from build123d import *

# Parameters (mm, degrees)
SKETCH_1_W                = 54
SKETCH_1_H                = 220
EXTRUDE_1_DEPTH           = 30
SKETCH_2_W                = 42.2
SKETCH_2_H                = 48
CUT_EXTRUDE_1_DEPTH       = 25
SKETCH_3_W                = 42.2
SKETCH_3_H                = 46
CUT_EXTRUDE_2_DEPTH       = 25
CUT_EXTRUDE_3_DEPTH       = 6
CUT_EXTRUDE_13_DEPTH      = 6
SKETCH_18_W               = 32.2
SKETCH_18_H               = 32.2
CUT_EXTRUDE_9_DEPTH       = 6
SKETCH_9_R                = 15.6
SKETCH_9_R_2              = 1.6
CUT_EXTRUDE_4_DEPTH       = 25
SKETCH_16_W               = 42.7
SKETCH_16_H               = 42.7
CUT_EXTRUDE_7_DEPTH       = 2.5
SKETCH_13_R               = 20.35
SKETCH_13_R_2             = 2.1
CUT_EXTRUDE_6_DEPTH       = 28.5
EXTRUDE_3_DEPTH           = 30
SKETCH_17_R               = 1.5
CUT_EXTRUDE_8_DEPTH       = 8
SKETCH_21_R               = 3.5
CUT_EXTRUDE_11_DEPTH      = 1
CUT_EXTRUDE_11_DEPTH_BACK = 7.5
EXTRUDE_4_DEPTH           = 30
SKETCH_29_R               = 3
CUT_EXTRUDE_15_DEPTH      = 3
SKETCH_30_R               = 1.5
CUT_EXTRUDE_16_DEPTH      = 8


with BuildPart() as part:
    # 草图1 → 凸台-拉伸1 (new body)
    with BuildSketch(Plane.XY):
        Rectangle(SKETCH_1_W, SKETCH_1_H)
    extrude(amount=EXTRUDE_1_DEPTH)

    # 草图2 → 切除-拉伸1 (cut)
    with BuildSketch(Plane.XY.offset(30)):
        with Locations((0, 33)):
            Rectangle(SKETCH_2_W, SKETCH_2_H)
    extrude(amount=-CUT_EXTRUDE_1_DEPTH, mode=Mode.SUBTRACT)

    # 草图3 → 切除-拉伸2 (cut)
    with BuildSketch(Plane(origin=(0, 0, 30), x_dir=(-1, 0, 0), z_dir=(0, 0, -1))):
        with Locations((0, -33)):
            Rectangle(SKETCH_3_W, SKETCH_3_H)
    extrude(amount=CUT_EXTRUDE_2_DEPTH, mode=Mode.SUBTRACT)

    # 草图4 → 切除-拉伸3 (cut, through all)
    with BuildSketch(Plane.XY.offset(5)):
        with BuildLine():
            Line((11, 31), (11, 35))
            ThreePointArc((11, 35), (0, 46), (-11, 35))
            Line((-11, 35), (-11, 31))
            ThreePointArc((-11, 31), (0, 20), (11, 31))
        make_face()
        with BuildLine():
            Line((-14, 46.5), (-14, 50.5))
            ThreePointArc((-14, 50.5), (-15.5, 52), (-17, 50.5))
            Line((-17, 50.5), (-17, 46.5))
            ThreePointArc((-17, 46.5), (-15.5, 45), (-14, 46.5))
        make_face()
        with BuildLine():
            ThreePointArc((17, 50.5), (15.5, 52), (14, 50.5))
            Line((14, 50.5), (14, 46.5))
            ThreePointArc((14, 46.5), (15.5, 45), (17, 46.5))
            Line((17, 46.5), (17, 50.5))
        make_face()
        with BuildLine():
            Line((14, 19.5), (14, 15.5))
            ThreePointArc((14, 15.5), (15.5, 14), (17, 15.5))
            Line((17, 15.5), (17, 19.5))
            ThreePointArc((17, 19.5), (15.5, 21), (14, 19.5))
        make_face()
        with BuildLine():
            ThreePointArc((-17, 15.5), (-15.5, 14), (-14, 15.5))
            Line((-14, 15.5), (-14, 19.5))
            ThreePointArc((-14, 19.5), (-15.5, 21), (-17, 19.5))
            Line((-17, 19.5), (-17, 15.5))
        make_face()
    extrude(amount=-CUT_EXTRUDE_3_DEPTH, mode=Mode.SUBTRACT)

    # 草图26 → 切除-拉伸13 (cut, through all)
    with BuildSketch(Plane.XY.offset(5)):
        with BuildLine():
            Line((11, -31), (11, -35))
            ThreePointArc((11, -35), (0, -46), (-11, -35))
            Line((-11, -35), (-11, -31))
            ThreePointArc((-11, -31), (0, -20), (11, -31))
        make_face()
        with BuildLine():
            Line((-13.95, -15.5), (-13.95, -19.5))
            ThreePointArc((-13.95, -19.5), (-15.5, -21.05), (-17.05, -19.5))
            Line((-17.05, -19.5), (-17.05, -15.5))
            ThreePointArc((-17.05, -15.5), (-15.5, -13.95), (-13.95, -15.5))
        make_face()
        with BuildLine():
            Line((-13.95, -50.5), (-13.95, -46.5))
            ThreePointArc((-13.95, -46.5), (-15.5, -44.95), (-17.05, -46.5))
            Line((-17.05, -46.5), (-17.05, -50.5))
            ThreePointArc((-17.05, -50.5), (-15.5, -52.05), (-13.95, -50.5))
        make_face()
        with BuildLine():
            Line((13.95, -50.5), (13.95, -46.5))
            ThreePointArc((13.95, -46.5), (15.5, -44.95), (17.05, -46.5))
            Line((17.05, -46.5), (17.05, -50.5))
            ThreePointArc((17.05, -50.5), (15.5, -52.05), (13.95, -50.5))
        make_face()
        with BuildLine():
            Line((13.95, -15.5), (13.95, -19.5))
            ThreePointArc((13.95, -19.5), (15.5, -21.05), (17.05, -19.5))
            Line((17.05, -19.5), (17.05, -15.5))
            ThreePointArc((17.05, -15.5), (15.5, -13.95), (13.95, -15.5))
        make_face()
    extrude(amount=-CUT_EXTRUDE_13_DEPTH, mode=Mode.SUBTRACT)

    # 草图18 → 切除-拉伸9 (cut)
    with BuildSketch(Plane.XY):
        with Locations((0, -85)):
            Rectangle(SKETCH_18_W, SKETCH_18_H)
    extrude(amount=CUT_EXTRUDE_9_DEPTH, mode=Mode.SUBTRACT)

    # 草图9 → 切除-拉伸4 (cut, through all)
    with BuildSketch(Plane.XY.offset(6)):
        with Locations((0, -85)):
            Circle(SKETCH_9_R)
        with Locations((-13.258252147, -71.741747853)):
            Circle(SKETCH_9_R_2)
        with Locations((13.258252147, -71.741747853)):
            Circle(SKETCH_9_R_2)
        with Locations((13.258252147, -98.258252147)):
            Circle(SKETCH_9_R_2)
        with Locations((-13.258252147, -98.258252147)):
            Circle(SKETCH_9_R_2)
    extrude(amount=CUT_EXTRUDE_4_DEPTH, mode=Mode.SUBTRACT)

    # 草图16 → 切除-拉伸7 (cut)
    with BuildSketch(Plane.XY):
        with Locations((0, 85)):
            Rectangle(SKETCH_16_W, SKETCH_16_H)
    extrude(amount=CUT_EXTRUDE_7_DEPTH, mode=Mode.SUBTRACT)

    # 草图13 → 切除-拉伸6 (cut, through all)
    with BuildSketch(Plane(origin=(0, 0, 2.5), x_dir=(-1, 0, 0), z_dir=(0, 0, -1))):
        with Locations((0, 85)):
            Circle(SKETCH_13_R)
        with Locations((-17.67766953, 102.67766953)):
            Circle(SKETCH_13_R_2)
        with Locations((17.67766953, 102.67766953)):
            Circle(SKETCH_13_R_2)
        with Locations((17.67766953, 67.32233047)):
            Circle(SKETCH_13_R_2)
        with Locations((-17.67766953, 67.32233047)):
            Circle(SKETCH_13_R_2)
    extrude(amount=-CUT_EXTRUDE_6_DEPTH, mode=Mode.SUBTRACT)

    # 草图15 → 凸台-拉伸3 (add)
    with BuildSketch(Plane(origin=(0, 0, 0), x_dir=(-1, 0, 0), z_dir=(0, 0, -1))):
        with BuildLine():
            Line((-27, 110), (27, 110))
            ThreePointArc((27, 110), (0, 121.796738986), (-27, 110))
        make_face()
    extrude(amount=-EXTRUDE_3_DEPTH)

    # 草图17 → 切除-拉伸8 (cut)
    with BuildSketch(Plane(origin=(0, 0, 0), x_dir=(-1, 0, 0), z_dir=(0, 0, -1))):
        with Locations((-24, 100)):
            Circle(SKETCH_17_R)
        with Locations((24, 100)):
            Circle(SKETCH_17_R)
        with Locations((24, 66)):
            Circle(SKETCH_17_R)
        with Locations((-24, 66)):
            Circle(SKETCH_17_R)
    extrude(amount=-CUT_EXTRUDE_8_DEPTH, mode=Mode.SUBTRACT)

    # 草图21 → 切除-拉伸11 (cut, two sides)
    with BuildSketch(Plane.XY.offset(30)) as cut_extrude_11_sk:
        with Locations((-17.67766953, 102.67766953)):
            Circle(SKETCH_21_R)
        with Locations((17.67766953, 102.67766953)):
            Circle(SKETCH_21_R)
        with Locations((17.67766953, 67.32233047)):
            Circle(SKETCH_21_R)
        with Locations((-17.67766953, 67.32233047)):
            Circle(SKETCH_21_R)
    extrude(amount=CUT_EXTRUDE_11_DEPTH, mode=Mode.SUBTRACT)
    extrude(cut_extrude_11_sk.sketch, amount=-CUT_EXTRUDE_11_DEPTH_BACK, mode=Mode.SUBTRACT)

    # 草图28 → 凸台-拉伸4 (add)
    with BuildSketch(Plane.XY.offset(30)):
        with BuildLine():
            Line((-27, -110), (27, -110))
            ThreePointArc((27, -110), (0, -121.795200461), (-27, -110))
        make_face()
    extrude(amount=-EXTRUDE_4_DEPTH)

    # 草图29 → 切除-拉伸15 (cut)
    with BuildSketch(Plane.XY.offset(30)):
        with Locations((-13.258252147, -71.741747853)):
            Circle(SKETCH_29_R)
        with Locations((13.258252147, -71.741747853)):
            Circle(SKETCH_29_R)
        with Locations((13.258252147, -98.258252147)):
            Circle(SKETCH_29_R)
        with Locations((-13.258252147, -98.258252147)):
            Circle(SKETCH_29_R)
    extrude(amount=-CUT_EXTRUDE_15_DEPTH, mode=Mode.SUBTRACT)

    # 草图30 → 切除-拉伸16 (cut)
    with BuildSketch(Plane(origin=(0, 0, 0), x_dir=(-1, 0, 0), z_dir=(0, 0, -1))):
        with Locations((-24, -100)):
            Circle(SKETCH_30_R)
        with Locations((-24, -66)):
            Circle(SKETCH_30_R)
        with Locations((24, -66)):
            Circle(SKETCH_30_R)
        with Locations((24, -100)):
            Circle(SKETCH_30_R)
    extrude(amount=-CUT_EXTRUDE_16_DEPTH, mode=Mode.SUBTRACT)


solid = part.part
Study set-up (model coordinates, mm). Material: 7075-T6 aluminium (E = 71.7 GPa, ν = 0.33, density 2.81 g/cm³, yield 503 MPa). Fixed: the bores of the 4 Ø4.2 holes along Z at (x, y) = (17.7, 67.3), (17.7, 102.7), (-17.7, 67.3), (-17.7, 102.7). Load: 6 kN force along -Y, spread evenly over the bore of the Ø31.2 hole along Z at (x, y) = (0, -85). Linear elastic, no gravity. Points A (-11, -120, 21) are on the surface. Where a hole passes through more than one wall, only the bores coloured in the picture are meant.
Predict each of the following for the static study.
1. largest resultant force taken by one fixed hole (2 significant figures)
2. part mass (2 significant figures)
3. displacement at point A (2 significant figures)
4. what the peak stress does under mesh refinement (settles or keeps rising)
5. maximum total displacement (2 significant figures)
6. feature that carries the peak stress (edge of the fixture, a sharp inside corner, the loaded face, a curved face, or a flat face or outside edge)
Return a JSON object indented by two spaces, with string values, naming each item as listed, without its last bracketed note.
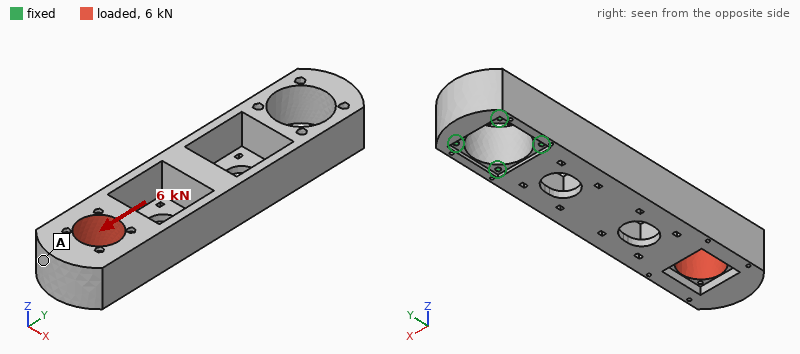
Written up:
{
  "largest resultant force taken by one fixed hole": "2.4 kN",
  "part mass": "590 g",
  "displacement at point A": "0.22 mm",
  "what the peak stress does under mesh refinement": "keeps rising",
  "maximum total displacement": "0.23 mm",
  "feature that carries the peak stress": "edge of the fixture"
}
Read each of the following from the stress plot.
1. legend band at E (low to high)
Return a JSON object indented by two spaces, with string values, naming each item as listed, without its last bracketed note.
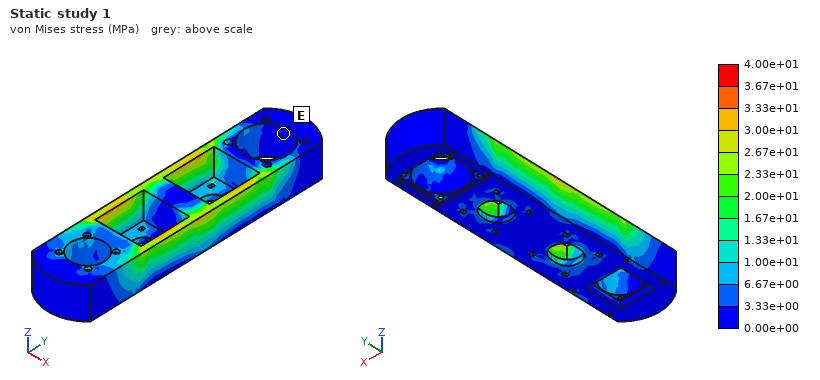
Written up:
{
  "legend band at E": "0.00e+00 to 3.33e+00 MPa"
}
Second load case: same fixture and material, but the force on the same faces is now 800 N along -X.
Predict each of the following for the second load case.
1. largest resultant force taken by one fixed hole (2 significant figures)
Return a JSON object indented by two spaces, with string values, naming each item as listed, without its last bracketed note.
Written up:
{
  "largest resultant force taken by one fixed hole": "2.5 kN"
}
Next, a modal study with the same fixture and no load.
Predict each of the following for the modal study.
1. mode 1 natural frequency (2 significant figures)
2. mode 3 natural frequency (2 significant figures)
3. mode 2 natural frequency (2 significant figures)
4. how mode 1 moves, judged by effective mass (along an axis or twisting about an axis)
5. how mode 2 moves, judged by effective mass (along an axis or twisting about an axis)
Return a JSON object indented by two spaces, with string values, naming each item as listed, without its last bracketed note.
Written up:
{
  "mode 1 natural frequency": "460 Hz",
  "mode 3 natural frequency": "1800 Hz",
  "mode 2 natural frequency": "780 Hz",
  "how mode 1 moves, judged by effective mass": "along Z",
  "how mode 2 moves, judged by effective mass": "along X"
}
